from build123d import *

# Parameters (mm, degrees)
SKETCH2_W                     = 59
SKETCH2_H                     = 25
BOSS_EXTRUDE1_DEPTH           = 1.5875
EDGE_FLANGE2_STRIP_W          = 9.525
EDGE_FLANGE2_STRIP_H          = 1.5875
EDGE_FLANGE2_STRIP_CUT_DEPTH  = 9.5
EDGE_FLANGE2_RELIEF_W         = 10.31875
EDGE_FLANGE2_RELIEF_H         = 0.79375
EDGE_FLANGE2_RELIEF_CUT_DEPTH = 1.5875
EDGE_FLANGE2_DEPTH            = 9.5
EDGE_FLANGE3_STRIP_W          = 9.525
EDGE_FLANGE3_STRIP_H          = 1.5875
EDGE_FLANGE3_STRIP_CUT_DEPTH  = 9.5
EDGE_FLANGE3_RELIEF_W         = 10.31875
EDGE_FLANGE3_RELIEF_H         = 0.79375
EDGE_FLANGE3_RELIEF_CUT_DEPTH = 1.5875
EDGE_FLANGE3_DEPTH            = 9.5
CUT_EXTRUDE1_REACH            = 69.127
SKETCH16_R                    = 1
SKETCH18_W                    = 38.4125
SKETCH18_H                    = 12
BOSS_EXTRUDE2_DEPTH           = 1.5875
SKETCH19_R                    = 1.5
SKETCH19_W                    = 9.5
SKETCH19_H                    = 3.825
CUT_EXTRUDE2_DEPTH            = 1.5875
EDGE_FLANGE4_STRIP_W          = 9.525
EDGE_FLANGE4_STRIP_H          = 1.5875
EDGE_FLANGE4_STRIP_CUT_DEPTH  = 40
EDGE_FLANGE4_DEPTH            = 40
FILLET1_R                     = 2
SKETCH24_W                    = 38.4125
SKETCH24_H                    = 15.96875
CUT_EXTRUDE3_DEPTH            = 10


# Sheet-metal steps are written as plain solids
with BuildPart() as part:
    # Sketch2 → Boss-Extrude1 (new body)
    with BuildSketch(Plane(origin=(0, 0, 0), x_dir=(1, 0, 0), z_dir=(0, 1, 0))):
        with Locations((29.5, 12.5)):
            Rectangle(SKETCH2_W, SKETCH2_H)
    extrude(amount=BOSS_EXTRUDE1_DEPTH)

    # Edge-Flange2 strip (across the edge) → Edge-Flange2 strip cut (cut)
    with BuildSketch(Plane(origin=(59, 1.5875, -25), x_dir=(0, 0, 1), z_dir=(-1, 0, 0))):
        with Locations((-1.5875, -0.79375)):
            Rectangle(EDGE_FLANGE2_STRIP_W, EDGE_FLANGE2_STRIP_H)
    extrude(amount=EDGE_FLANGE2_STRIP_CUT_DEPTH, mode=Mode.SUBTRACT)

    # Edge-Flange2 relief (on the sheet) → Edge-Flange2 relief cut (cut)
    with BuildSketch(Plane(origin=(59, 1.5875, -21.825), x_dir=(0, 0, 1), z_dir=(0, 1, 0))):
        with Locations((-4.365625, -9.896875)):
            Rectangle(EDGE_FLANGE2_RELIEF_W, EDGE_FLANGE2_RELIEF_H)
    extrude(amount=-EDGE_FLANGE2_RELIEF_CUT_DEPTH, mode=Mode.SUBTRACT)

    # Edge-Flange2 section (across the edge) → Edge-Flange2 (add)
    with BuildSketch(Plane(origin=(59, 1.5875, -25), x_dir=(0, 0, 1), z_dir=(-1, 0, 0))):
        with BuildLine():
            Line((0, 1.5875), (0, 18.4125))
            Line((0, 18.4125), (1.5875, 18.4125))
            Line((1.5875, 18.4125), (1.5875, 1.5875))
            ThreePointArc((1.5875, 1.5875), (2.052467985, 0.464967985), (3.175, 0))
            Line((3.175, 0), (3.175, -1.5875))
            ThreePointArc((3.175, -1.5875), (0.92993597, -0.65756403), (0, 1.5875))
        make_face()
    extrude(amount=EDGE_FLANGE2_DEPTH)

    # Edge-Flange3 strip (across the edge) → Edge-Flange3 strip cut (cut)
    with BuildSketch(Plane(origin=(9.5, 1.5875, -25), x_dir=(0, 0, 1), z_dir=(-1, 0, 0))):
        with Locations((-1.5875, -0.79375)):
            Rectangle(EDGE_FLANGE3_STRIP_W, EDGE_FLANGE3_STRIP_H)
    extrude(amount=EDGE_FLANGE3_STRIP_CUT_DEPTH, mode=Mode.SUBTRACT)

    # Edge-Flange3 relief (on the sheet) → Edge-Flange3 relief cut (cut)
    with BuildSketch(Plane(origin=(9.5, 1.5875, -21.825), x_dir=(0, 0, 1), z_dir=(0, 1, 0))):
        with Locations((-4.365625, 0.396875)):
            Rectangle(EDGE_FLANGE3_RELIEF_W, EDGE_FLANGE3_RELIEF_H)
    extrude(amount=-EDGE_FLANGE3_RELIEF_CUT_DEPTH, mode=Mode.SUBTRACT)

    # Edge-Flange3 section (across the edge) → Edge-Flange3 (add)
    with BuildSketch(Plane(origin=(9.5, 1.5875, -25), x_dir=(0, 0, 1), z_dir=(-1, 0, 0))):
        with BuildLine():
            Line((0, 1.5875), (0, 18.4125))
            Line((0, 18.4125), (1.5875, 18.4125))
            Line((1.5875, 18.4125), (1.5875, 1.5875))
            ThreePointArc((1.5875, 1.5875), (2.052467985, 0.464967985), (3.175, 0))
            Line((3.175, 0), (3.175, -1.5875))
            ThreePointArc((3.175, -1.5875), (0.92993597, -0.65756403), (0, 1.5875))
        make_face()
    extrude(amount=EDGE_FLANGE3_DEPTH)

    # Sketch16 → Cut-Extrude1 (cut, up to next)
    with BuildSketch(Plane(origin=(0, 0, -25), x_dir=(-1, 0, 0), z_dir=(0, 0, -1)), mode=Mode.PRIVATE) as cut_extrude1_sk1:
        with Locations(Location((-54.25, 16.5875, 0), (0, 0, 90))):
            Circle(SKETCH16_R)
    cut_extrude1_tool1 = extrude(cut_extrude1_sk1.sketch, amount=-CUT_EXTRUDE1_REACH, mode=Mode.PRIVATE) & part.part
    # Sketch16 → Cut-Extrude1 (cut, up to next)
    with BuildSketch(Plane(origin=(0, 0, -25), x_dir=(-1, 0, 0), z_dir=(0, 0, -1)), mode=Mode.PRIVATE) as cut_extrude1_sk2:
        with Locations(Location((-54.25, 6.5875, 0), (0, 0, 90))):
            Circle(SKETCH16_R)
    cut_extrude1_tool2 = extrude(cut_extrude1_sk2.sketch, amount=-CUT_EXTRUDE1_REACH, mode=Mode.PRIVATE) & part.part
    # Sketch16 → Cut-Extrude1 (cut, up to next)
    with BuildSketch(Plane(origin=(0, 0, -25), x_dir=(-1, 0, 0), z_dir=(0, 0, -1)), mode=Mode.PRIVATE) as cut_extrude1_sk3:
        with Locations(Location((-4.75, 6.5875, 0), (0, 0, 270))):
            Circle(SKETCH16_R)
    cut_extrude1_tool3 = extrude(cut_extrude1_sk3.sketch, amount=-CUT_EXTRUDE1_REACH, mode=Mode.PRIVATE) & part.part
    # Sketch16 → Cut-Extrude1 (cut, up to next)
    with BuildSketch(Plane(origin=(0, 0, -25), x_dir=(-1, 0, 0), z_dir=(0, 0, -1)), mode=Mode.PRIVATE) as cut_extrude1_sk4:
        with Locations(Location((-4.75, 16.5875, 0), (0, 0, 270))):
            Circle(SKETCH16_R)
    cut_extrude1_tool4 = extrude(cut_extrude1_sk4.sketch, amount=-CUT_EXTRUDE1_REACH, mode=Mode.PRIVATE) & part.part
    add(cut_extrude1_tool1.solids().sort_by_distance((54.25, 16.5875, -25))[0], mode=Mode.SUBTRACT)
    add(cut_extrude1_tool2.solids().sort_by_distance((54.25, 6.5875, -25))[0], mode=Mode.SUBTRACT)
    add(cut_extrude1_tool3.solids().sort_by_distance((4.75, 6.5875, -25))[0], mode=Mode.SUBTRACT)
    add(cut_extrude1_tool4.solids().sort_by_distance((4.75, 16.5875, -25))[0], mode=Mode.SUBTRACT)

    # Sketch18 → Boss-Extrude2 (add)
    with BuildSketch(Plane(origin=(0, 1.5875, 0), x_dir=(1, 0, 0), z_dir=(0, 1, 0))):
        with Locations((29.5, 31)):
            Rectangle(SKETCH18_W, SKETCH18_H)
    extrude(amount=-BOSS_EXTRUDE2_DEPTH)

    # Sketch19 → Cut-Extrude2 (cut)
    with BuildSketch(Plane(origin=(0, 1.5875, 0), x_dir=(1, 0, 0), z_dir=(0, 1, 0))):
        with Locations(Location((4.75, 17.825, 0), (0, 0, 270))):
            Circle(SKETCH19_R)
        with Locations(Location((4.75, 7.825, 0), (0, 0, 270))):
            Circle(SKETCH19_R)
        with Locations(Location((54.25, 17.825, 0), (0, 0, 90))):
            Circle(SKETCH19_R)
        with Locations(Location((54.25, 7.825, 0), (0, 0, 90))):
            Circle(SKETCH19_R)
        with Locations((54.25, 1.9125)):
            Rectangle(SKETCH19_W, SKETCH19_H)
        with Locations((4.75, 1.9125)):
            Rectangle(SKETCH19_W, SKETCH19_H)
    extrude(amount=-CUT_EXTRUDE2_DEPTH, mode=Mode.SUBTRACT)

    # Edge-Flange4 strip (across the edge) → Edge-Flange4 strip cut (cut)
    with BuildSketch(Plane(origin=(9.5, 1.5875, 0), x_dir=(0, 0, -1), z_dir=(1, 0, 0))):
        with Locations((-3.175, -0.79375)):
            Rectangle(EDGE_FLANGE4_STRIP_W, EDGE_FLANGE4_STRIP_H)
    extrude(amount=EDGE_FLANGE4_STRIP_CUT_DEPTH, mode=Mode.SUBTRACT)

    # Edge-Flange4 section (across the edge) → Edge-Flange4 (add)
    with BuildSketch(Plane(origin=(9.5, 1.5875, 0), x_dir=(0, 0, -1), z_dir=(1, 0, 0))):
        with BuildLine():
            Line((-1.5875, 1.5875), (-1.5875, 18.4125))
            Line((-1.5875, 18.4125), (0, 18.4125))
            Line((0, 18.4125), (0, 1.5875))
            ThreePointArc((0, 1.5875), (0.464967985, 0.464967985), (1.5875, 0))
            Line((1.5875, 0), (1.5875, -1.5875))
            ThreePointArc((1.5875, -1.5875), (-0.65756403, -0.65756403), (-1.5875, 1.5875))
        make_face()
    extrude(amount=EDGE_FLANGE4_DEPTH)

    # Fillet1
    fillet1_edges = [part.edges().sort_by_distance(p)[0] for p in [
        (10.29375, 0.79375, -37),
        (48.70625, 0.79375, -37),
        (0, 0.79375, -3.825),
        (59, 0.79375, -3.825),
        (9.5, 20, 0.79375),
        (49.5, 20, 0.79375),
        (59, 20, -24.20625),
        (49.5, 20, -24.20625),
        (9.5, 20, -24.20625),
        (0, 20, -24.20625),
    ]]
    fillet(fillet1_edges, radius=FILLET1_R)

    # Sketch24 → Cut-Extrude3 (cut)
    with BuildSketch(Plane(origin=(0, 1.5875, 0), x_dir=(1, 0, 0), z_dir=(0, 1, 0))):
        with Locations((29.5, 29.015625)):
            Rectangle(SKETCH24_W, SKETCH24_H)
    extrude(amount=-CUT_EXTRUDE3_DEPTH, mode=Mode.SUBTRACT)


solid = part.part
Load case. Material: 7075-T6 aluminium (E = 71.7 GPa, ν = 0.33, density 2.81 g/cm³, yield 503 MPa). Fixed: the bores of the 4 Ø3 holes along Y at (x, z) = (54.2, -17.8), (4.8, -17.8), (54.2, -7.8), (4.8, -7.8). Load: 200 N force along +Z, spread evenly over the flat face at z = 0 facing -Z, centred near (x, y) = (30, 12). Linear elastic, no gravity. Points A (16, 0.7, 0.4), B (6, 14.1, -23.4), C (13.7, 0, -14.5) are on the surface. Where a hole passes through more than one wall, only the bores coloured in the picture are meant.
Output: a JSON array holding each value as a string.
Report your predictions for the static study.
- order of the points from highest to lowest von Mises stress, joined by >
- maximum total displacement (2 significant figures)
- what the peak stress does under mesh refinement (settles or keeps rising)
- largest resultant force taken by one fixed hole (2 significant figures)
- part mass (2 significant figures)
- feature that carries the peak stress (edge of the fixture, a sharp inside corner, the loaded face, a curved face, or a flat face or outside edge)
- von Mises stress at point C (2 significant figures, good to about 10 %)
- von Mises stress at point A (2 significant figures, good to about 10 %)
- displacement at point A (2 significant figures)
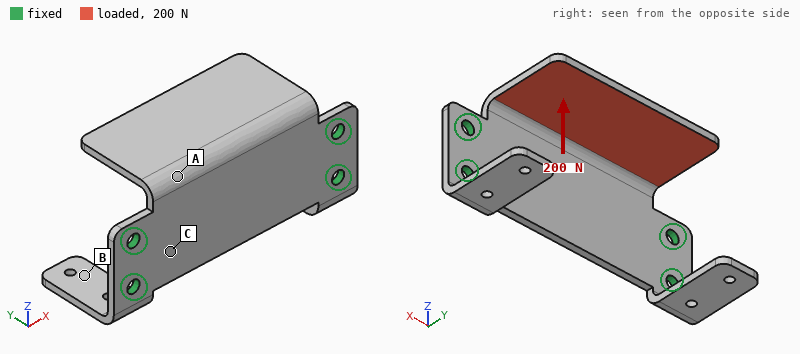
["A > C > B", "0.69 mm", "keeps rising", "120 N", "10 g", "a sharp inside corner", "39 MPa", "94 MPa", "0.14 mm"]
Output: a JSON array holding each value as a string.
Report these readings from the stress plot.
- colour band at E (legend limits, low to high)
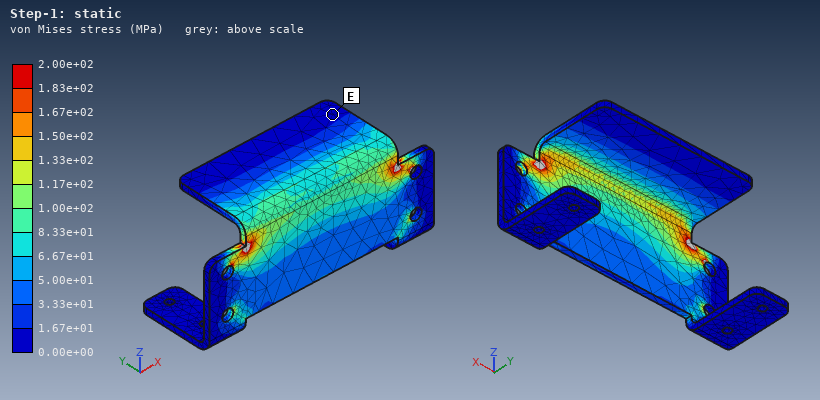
["0.00e+00 to 1.67e+01 MPa"]
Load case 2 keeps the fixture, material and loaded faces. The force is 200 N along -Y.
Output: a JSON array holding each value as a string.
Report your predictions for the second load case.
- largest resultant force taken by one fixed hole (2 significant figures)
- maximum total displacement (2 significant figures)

["150 N", "0.27 mm"]
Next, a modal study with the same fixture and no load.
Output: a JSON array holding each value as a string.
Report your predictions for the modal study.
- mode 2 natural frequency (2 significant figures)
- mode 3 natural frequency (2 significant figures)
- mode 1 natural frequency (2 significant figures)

["2600 Hz", "2600 Hz", "1800 Hz"]
